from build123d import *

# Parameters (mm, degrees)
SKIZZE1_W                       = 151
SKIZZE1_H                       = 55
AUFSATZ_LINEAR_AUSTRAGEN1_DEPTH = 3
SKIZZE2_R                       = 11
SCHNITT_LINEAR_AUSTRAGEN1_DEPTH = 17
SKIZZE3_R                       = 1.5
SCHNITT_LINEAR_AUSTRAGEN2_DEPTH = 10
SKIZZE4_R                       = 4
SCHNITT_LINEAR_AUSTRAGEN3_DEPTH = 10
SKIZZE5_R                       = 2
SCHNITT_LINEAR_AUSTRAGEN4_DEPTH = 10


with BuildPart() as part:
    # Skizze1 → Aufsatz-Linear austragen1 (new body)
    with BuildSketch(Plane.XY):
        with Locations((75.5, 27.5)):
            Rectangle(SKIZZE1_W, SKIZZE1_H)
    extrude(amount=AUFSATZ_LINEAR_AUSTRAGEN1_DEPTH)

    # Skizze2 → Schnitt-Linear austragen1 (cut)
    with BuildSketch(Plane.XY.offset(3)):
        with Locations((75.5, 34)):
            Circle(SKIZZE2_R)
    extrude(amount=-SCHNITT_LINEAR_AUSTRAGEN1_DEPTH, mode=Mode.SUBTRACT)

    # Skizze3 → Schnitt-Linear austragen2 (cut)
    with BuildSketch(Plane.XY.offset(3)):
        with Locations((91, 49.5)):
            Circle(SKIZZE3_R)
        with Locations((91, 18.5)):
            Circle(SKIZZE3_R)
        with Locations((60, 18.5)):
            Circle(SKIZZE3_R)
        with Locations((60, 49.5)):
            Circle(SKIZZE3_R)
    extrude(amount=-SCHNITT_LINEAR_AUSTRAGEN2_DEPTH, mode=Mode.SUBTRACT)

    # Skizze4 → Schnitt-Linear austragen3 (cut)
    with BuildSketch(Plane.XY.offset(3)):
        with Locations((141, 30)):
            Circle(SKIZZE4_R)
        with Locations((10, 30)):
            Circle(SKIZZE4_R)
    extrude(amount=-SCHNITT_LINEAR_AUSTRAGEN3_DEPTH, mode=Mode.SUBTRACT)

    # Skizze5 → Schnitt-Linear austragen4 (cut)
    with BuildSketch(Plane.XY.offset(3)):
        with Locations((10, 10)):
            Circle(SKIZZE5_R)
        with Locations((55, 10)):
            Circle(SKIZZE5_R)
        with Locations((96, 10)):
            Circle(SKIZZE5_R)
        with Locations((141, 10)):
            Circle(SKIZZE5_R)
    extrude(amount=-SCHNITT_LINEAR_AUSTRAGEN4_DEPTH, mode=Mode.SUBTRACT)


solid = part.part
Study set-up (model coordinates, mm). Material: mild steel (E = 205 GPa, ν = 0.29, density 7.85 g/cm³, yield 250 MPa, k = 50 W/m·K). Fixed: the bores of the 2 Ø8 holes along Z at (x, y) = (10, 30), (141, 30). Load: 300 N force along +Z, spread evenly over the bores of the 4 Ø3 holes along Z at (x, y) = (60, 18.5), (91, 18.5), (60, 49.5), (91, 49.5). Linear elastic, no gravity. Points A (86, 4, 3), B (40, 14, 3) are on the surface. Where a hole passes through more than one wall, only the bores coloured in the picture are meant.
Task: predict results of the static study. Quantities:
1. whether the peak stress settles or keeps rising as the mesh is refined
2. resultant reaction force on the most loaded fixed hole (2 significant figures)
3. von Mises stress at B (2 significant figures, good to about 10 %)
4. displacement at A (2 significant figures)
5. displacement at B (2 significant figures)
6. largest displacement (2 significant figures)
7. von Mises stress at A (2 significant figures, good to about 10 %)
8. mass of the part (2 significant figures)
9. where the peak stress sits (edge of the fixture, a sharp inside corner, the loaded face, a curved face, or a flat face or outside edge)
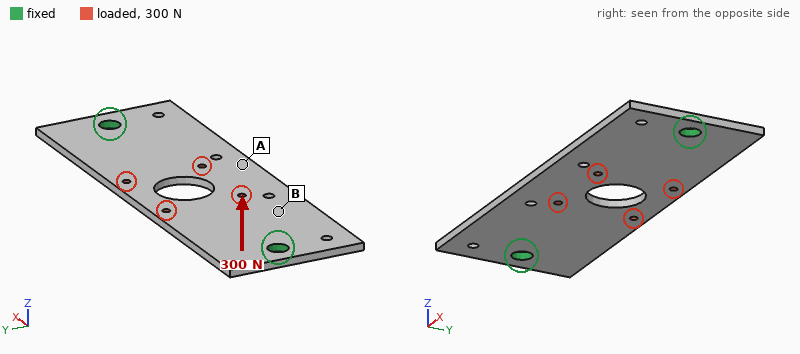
keeps rising
150 N
10 MPa
0.11 mm
0.059 mm
0.18 mm
35 MPa
180 g
edge of the fixture
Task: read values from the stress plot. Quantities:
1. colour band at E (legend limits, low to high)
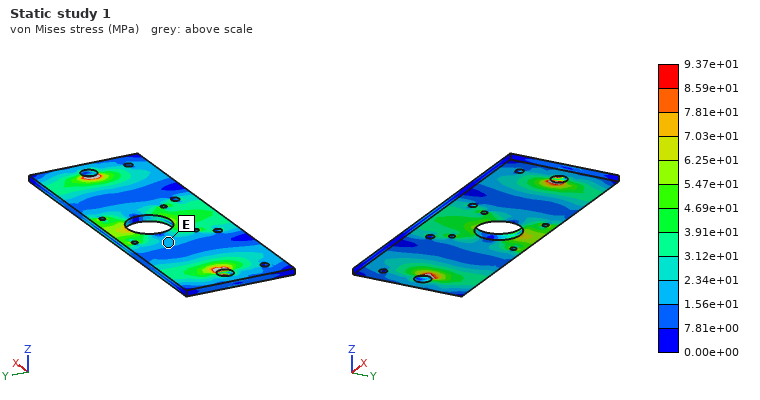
1.56e+01 to 2.34e+01 MPa
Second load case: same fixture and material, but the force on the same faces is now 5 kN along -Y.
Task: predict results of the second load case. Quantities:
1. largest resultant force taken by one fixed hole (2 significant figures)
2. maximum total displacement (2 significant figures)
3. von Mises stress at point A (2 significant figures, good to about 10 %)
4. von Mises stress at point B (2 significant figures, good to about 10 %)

2.6 kN
33 µm
61 MPa
34 MPa
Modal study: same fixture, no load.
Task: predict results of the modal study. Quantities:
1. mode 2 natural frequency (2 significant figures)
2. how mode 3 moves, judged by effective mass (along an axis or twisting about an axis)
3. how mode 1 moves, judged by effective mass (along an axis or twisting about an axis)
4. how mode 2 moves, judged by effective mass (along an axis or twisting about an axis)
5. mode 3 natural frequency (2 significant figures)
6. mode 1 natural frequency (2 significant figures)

1300 Hz
twisting about Y
along Z
twisting about X
2200 Hz
890 Hz
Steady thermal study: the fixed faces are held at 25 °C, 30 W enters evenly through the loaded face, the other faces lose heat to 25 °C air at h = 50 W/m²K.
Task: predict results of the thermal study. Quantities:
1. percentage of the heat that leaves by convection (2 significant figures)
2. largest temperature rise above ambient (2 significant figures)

69 %
68 K
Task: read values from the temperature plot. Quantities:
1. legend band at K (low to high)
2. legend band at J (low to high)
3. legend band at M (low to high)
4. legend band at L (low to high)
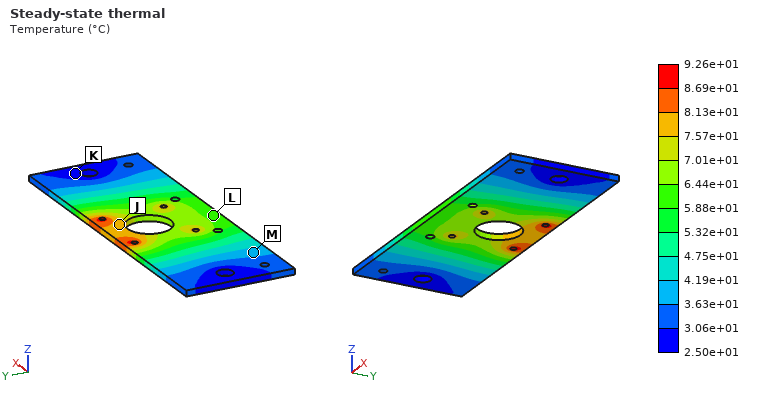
2.50e+01 to 3.06e+01 °C
7.57e+01 to 8.13e+01 °C
3.63e+01 to 4.19e+01 °C
5.88e+01 to 6.44e+01 °C
